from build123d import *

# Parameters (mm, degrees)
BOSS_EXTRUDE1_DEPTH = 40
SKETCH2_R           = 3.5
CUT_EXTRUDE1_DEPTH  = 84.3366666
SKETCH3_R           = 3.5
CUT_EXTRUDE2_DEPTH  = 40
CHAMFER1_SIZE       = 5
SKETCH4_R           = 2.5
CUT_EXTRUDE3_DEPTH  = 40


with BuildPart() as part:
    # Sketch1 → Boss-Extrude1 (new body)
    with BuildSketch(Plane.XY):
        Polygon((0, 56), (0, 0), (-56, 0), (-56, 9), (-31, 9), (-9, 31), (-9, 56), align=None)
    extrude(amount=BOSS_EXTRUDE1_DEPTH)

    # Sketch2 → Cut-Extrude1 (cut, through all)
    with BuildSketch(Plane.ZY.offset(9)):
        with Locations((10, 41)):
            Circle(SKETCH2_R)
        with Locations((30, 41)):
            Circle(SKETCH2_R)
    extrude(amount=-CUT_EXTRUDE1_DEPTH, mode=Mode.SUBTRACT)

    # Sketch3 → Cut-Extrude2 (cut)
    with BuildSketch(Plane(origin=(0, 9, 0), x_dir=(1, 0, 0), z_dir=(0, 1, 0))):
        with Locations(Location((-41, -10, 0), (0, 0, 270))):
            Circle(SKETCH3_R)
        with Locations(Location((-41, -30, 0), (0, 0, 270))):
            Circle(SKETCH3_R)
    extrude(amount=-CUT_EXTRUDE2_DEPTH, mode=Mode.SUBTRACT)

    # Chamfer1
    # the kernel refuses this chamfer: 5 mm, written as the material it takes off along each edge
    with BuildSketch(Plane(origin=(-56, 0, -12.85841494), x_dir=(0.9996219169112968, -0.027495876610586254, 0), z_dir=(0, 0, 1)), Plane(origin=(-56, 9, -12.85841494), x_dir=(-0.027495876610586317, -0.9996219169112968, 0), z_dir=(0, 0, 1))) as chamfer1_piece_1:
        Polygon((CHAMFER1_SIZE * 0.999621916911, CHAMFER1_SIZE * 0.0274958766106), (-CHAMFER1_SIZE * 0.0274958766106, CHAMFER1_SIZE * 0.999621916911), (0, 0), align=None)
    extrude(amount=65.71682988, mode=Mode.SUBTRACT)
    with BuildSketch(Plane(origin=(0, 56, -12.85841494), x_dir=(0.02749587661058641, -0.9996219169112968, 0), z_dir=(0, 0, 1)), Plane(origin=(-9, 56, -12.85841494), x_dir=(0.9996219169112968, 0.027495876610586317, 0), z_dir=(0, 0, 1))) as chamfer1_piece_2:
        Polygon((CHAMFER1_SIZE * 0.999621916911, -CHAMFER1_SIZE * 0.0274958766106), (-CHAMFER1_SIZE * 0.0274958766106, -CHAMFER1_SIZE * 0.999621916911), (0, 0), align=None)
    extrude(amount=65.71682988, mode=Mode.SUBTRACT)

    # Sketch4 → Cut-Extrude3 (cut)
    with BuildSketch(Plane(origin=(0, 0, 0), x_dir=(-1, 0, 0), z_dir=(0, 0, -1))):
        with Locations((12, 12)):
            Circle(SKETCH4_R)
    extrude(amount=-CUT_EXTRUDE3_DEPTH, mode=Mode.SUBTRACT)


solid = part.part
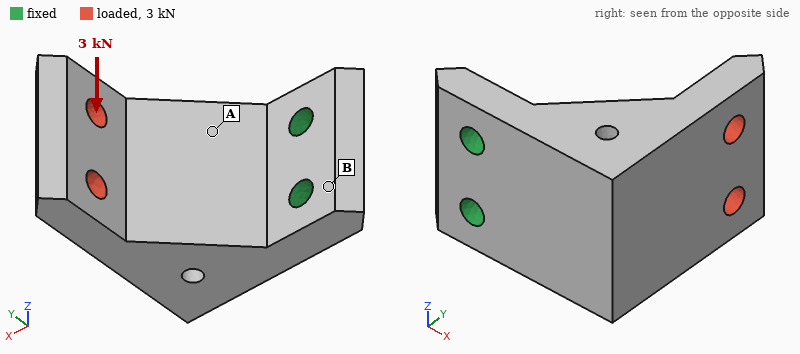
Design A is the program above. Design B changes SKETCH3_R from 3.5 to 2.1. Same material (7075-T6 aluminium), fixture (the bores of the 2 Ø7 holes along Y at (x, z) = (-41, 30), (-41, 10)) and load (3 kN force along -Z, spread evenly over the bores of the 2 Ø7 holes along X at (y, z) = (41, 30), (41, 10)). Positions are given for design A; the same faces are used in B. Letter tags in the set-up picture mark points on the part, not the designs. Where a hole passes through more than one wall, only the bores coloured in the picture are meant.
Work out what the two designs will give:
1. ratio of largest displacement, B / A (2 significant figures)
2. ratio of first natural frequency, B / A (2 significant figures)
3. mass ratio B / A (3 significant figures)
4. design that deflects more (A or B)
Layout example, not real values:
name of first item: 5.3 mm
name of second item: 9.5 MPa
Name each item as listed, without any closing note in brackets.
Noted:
ratio of largest displacement, B / A: 1.2
ratio of first natural frequency, B / A: 0.90
mass ratio B / A: 1.01
design that deflects more: B
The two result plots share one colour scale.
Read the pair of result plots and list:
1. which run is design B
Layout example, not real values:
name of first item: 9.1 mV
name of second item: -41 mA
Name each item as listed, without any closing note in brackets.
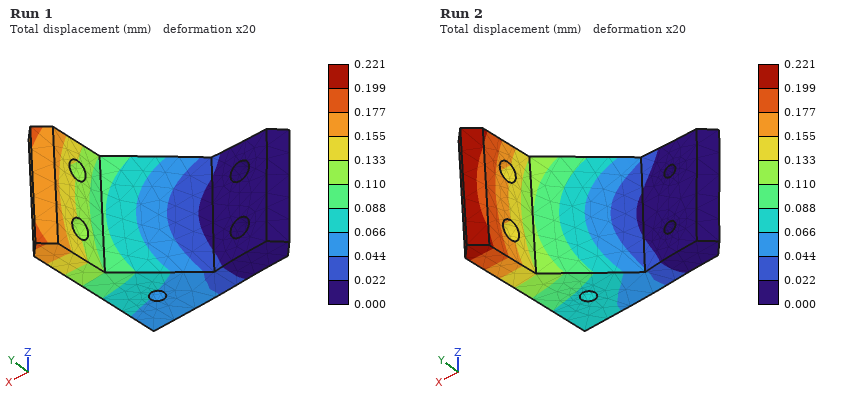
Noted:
which run is design B: Run 2
